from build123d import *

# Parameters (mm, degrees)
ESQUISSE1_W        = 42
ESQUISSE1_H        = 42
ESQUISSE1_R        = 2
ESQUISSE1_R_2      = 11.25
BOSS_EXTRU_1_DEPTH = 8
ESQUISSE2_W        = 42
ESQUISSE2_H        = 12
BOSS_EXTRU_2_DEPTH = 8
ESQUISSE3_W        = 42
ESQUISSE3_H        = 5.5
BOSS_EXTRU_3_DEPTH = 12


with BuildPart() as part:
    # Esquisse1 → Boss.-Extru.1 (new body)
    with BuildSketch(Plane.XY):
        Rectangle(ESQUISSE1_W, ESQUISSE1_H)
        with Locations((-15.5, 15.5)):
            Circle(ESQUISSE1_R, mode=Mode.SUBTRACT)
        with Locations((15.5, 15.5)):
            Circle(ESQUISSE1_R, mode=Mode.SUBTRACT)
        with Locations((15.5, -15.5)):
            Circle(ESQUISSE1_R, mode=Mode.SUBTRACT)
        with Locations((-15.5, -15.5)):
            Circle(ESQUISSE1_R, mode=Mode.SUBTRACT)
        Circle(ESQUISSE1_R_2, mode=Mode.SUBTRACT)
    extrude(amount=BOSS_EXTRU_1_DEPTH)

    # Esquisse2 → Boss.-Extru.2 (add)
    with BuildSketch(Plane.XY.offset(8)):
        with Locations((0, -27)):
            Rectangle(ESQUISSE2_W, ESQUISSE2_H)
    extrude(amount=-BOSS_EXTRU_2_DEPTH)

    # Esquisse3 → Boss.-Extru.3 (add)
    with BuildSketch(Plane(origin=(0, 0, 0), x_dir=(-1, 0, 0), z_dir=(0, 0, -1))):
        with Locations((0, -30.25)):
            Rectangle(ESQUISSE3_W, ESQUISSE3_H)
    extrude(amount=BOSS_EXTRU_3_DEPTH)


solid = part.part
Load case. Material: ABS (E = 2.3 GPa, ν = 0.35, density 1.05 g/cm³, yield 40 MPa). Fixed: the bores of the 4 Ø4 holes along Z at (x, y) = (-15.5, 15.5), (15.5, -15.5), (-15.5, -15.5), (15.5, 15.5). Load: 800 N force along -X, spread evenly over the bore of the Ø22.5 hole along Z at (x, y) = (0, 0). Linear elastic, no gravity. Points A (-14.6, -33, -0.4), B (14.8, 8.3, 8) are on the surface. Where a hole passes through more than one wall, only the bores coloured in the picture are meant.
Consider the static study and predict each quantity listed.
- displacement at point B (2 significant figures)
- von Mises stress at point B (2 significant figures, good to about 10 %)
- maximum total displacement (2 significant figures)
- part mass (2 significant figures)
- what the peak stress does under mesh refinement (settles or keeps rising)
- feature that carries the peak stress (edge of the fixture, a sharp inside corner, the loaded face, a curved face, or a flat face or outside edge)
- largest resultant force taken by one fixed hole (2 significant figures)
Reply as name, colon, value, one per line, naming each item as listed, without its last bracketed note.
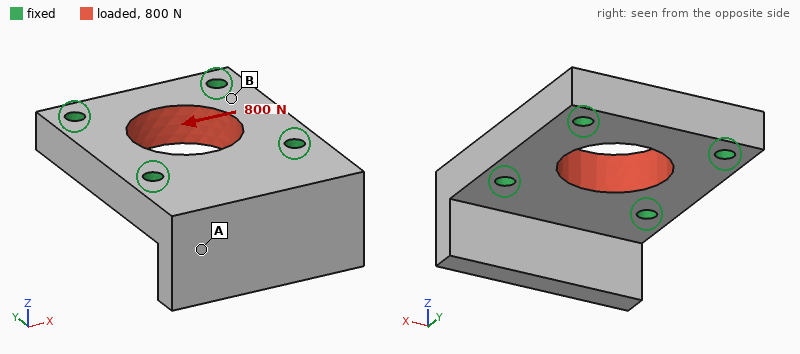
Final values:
displacement at point B: 14 µm
von Mises stress at point B: 2.0 MPa
maximum total displacement: 27 µm
part mass: 18 g
what the peak stress does under mesh refinement: keeps rising
feature that carries the peak stress: edge of the fixture
largest resultant force taken by one fixed hole: 210 N
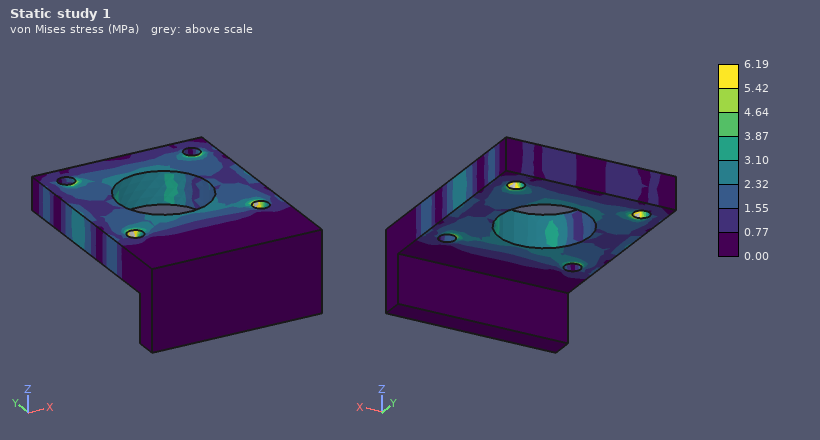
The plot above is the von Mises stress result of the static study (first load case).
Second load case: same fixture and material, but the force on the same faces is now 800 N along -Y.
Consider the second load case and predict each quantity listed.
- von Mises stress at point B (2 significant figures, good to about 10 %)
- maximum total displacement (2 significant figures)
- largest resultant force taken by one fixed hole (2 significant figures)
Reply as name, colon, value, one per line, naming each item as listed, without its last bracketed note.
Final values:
von Mises stress at point B: 1.7 MPa
maximum total displacement: 29 µm
largest resultant force taken by one fixed hole: 210 N
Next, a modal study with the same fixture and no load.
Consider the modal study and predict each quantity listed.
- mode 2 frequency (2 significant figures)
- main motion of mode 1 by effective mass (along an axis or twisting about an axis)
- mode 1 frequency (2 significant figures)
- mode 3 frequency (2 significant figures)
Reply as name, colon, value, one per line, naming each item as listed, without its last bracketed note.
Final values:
mode 2 frequency: 4100 Hz
main motion of mode 1 by effective mass: along Z
mode 1 frequency: 2600 Hz
mode 3 frequency: 5900 Hz
